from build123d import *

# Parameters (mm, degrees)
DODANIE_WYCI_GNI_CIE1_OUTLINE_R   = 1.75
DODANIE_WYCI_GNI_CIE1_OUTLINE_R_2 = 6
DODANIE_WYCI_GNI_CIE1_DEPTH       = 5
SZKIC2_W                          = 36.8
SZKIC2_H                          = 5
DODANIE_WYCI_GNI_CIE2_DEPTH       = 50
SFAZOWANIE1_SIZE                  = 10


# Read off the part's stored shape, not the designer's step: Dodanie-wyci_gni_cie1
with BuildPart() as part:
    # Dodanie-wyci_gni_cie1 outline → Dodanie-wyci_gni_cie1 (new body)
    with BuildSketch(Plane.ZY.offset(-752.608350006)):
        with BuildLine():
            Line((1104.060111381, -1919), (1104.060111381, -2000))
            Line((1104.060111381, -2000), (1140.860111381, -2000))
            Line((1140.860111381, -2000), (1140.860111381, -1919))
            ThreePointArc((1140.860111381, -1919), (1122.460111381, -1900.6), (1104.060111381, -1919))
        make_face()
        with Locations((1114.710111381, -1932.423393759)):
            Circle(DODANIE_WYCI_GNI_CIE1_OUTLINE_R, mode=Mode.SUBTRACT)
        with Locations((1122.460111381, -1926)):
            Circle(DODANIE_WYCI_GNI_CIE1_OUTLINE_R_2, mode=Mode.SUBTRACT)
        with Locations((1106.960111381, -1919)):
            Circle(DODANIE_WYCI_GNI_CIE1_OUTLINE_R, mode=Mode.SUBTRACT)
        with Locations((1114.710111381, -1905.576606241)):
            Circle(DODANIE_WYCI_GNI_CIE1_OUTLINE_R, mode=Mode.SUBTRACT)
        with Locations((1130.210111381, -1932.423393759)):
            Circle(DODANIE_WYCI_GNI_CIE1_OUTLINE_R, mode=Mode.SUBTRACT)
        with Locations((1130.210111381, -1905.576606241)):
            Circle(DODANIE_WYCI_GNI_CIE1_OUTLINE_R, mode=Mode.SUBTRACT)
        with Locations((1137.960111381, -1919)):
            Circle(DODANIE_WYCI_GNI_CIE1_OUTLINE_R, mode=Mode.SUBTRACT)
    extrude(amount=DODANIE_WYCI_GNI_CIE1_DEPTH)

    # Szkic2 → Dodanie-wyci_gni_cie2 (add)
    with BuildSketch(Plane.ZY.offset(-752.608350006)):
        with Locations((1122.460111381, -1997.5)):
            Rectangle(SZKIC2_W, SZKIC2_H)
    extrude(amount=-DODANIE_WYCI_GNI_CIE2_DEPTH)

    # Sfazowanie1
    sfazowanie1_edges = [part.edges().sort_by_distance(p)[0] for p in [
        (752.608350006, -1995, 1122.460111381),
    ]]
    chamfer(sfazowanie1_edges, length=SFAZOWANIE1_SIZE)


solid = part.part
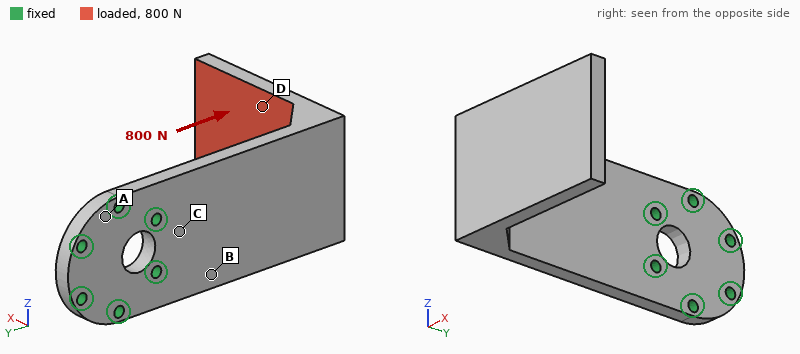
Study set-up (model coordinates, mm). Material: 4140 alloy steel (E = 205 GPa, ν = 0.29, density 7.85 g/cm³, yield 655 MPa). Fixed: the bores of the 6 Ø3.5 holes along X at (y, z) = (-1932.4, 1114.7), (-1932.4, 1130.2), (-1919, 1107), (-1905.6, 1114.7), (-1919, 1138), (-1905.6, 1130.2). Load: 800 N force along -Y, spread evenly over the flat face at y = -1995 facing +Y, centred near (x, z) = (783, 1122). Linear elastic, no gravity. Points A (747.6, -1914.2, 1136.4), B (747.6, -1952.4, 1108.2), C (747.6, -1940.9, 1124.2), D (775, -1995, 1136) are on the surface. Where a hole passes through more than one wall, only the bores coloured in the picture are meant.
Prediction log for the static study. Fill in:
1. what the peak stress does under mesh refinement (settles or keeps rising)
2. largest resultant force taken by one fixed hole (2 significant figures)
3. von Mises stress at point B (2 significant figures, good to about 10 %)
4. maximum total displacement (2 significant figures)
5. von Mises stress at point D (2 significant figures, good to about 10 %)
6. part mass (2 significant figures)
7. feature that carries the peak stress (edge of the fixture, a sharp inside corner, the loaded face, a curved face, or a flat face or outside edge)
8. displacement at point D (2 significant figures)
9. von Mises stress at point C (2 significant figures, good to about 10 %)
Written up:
keeps rising
440 N
160 MPa
1.3 mm
49 MPa
220 g
edge of the fixture
0.79 mm
150 MPa
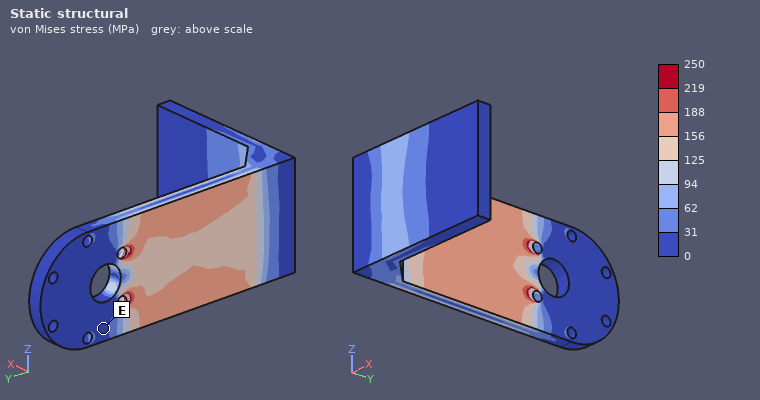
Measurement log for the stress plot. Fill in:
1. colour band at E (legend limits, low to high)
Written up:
0 to 31 MPa
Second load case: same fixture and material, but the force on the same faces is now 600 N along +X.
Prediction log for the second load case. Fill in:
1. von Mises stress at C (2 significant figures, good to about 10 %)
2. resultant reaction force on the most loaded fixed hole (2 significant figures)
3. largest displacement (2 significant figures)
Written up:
190 MPa
700 N
1.0 mm
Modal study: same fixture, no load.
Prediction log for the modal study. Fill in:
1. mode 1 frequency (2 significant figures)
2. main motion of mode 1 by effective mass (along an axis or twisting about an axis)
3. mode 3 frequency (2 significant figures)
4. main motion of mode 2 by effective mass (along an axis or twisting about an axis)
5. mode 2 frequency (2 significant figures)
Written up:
380 Hz
along X
1500 Hz
along Z
860 Hz
